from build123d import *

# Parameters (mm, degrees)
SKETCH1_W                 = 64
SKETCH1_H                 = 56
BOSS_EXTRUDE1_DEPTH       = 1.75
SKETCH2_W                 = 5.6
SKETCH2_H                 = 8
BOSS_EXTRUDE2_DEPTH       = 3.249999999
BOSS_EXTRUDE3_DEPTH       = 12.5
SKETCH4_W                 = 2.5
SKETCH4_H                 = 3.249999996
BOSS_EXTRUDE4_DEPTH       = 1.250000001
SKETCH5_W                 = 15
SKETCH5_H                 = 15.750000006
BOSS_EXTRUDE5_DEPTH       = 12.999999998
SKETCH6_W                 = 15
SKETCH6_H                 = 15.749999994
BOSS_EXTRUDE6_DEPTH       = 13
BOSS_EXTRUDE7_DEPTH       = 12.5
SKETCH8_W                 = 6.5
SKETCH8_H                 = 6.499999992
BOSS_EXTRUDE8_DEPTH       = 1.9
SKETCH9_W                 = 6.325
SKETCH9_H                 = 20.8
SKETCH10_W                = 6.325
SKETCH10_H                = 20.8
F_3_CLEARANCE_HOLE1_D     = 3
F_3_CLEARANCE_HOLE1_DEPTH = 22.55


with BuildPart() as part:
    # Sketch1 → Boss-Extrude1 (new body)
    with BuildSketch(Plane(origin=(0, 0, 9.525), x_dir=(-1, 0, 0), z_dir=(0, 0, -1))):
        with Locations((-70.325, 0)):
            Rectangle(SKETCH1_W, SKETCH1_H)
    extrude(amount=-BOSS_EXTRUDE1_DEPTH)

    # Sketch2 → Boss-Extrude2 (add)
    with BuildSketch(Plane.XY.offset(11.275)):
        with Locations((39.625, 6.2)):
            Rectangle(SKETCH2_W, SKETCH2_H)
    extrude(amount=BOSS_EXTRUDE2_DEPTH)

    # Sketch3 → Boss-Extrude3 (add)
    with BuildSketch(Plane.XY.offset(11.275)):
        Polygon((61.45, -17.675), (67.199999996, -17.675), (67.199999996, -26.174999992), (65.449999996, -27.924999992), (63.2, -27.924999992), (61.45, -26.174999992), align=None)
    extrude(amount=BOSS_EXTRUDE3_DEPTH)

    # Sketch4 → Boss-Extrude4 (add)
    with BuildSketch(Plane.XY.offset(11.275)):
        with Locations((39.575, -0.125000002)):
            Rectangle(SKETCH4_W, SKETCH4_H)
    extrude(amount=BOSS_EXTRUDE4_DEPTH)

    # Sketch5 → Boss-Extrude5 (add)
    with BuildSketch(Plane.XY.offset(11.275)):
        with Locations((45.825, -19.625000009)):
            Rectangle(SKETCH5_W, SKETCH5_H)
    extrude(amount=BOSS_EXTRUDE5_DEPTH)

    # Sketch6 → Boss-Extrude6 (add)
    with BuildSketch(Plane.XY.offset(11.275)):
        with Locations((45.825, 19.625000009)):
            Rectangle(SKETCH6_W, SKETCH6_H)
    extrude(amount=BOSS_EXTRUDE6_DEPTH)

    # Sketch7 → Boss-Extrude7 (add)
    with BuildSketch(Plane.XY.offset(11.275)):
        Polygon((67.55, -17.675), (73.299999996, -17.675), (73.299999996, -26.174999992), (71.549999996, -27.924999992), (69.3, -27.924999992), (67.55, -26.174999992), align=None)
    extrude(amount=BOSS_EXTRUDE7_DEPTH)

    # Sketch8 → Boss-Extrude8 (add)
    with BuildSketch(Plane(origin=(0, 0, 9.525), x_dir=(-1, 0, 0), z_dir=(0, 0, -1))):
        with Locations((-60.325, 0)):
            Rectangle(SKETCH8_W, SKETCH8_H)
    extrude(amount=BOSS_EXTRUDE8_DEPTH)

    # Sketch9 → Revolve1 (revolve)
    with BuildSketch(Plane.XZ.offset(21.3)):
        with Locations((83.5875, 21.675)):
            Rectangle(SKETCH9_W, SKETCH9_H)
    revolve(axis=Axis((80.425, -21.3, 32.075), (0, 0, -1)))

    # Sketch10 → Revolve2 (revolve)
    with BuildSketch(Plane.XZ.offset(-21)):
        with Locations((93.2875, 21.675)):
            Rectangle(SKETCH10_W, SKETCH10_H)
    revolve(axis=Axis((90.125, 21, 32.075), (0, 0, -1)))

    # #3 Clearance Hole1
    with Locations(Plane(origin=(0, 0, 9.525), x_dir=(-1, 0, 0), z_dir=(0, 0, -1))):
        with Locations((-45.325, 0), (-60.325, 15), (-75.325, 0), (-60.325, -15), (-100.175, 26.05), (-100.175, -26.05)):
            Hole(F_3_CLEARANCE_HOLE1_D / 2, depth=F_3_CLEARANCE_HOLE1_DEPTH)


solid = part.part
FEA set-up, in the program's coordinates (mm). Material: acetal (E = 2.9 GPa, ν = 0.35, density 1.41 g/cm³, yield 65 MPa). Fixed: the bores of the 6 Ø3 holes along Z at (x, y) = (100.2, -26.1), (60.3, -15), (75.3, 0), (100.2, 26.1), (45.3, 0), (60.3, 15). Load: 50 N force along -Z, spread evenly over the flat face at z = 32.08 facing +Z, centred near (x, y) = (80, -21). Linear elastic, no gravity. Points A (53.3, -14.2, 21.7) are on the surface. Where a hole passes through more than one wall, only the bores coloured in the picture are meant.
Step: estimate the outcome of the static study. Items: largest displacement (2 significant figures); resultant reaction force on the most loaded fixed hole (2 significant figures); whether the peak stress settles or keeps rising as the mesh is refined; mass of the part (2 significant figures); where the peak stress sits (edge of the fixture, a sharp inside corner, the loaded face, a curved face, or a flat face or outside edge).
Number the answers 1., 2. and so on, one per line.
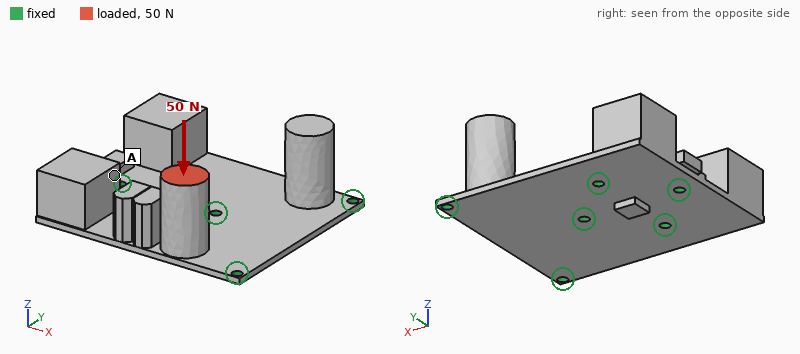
1. 0.59 mm
2. 26 N
3. keeps rising
4. 27 g
5. edge of the fixture
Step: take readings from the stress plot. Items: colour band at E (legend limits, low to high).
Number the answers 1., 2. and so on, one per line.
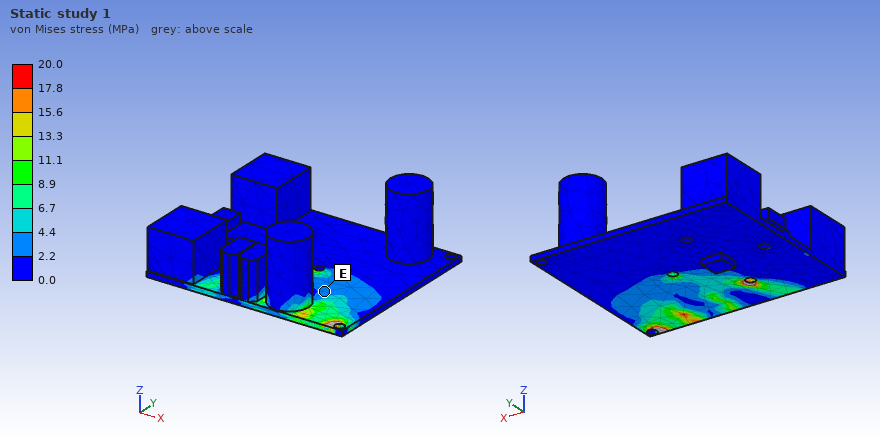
1. 2.2 to 4.4 MPa
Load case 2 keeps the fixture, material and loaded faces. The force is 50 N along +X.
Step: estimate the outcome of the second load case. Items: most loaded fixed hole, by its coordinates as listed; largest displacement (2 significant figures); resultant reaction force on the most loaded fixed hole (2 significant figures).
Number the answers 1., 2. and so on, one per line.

1. (60.3, -15)
2. 0.93 mm
3. 51 N
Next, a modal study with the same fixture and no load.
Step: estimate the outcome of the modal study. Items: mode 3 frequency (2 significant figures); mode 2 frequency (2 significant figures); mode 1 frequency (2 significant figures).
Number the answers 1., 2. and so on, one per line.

1. 590 Hz
2. 490 Hz
3. 470 Hz
